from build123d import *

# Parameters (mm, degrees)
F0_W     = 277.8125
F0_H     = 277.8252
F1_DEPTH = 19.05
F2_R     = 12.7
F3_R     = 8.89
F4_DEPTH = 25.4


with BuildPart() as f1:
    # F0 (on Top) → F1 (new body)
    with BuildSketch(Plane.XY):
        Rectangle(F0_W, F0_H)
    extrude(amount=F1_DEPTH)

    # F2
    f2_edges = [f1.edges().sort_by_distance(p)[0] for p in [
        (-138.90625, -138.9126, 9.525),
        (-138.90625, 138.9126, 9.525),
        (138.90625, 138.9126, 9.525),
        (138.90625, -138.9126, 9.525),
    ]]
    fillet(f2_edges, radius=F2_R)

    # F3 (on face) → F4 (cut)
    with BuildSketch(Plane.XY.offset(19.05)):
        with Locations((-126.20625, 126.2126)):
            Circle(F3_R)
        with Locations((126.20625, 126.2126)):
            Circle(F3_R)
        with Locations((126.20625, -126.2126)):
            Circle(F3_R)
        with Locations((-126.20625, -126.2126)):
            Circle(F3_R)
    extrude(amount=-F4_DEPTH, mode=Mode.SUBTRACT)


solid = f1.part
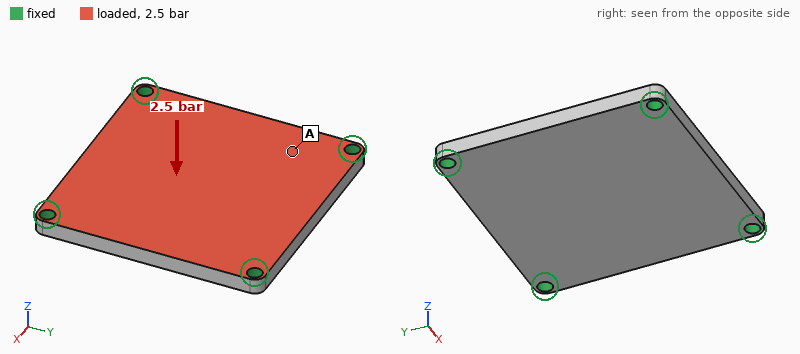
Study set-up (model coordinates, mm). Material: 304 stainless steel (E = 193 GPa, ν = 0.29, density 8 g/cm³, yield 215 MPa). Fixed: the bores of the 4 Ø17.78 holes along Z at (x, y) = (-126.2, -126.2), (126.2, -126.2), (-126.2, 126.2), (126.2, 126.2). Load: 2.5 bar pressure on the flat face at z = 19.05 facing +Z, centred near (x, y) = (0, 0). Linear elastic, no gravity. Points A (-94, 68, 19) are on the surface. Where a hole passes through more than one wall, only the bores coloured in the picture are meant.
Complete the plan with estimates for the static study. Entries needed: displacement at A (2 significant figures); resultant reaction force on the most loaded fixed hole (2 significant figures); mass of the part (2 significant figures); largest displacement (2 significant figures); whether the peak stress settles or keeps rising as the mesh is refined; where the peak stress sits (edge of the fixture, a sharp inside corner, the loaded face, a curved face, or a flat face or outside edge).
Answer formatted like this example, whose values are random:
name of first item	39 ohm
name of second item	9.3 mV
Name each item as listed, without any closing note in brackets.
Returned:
displacement at A	33 µm
resultant reaction force on the most loaded fixed hole	4.8 kN
mass of the part	12 kg
largest displacement	71 µm
whether the peak stress settles or keeps rising as the mesh is refined	keeps rising
where the peak stress sits	edge of the fixture
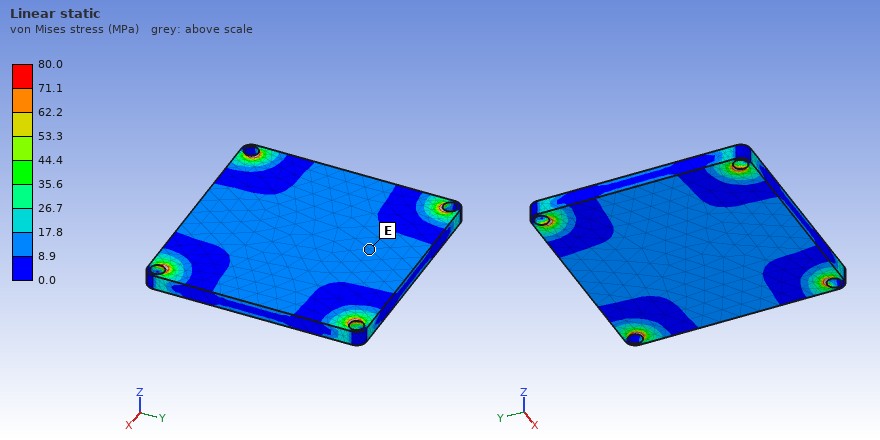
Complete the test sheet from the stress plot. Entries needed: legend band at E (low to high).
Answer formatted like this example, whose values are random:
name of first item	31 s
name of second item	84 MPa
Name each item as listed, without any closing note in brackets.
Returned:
legend band at E	8.9 to 17.8 MPa
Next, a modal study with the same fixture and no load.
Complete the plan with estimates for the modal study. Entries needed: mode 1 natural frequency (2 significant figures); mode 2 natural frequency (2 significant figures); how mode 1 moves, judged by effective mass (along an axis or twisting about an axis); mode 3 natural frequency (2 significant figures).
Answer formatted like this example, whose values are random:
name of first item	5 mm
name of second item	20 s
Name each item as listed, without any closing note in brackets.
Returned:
mode 1 natural frequency	920 Hz
mode 2 natural frequency	1600 Hz
how mode 1 moves, judged by effective mass	along Z
mode 3 natural frequency	1600 Hz
